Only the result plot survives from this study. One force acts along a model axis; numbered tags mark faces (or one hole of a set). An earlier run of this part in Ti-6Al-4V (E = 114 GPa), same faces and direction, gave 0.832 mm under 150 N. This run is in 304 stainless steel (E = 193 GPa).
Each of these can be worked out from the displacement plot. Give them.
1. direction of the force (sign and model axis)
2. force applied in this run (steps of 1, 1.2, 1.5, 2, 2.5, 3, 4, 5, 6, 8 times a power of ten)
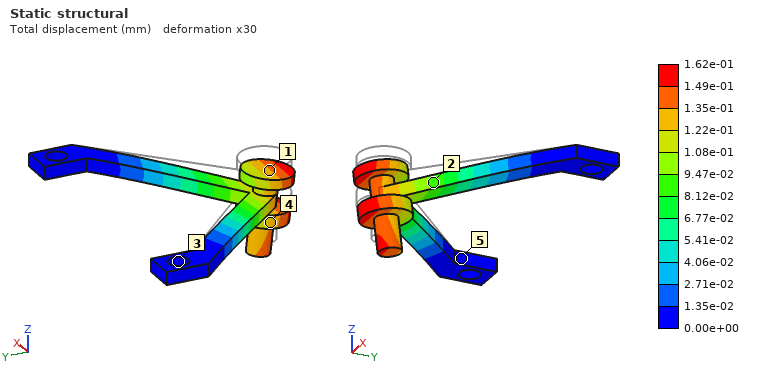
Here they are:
-Z
50 N
